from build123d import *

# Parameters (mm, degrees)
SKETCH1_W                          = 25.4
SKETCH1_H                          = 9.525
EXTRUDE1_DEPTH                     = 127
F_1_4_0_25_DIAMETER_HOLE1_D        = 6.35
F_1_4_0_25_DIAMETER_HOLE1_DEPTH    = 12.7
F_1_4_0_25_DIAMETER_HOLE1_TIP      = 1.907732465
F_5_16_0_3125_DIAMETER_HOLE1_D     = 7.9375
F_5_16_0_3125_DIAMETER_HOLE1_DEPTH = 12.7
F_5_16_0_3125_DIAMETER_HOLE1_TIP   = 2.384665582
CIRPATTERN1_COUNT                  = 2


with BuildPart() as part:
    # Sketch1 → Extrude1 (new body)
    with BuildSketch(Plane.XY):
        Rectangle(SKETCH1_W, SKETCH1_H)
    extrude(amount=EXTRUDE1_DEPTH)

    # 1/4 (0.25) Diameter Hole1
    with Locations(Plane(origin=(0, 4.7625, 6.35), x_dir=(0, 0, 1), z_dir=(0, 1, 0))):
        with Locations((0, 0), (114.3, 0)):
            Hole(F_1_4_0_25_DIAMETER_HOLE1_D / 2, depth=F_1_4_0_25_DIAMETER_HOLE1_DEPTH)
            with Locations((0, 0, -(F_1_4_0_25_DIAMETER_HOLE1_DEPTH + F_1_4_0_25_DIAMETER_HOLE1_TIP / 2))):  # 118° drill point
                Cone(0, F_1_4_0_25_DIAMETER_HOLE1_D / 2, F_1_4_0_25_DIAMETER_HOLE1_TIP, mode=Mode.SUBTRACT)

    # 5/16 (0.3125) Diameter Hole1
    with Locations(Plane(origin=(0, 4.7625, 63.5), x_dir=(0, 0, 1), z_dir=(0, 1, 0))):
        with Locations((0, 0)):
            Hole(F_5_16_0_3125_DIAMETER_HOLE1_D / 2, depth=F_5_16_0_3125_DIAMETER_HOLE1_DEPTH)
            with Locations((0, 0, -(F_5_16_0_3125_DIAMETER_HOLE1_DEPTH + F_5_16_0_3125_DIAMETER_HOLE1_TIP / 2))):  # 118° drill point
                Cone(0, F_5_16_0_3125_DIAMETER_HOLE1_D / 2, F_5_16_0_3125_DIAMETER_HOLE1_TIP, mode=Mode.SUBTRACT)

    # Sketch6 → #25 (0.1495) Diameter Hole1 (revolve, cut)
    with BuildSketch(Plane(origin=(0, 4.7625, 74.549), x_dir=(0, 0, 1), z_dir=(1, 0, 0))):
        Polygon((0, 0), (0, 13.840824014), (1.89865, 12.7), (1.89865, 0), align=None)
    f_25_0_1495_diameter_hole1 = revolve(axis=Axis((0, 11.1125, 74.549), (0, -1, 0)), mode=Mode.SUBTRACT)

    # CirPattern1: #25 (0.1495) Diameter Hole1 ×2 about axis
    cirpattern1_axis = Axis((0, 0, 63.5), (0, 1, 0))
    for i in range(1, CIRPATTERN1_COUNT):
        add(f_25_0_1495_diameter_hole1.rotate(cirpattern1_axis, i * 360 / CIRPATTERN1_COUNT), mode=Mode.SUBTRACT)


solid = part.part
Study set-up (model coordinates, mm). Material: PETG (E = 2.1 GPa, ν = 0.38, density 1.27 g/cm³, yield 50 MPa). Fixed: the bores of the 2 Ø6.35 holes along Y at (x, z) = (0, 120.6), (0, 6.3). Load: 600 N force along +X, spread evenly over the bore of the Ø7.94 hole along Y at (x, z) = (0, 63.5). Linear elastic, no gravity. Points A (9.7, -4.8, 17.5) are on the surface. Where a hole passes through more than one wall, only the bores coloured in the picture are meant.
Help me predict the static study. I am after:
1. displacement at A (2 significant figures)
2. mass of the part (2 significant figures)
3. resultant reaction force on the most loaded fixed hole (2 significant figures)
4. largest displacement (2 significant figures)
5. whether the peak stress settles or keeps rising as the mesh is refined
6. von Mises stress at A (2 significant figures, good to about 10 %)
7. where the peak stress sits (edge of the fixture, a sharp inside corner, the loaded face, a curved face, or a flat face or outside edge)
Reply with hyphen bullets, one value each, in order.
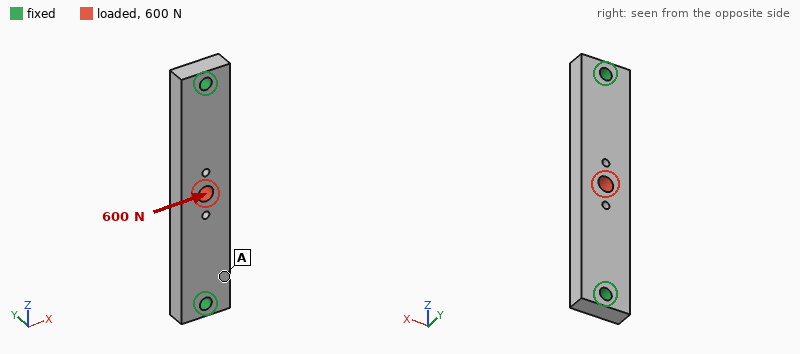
- 0.11 mm
- 37 g
- 300 N
- 0.44 mm
- keeps rising
- 2.2 MPa
- edge of the fixture
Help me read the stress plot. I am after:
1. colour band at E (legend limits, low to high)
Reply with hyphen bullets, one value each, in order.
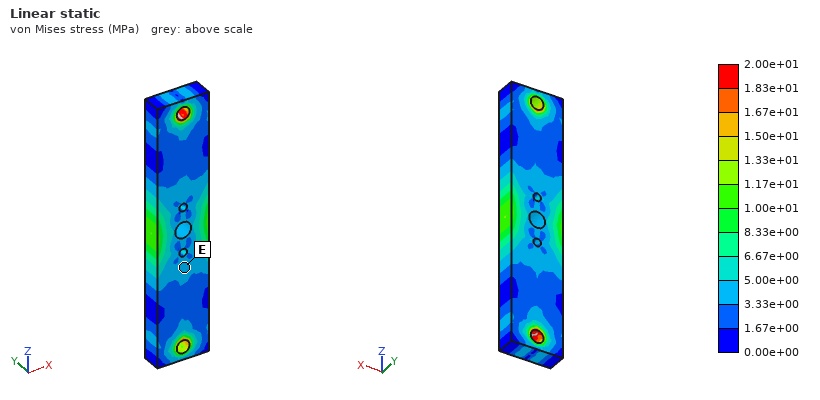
- 3.33e+00 to 5.00e+00 MPa
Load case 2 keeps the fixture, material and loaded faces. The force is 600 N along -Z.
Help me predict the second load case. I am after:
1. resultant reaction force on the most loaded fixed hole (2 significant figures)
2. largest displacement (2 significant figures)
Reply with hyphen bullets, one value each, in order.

- 300 N
- 43 µm
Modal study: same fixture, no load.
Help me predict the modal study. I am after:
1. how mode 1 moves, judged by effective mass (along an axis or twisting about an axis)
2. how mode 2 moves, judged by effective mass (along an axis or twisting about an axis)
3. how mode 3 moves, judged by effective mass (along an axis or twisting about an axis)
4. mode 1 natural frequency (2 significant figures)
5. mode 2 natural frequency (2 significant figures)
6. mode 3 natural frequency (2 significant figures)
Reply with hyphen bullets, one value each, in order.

- along Y
- along X
- twisting about Z
- 920 Hz
- 1500 Hz
- 2100 Hz
